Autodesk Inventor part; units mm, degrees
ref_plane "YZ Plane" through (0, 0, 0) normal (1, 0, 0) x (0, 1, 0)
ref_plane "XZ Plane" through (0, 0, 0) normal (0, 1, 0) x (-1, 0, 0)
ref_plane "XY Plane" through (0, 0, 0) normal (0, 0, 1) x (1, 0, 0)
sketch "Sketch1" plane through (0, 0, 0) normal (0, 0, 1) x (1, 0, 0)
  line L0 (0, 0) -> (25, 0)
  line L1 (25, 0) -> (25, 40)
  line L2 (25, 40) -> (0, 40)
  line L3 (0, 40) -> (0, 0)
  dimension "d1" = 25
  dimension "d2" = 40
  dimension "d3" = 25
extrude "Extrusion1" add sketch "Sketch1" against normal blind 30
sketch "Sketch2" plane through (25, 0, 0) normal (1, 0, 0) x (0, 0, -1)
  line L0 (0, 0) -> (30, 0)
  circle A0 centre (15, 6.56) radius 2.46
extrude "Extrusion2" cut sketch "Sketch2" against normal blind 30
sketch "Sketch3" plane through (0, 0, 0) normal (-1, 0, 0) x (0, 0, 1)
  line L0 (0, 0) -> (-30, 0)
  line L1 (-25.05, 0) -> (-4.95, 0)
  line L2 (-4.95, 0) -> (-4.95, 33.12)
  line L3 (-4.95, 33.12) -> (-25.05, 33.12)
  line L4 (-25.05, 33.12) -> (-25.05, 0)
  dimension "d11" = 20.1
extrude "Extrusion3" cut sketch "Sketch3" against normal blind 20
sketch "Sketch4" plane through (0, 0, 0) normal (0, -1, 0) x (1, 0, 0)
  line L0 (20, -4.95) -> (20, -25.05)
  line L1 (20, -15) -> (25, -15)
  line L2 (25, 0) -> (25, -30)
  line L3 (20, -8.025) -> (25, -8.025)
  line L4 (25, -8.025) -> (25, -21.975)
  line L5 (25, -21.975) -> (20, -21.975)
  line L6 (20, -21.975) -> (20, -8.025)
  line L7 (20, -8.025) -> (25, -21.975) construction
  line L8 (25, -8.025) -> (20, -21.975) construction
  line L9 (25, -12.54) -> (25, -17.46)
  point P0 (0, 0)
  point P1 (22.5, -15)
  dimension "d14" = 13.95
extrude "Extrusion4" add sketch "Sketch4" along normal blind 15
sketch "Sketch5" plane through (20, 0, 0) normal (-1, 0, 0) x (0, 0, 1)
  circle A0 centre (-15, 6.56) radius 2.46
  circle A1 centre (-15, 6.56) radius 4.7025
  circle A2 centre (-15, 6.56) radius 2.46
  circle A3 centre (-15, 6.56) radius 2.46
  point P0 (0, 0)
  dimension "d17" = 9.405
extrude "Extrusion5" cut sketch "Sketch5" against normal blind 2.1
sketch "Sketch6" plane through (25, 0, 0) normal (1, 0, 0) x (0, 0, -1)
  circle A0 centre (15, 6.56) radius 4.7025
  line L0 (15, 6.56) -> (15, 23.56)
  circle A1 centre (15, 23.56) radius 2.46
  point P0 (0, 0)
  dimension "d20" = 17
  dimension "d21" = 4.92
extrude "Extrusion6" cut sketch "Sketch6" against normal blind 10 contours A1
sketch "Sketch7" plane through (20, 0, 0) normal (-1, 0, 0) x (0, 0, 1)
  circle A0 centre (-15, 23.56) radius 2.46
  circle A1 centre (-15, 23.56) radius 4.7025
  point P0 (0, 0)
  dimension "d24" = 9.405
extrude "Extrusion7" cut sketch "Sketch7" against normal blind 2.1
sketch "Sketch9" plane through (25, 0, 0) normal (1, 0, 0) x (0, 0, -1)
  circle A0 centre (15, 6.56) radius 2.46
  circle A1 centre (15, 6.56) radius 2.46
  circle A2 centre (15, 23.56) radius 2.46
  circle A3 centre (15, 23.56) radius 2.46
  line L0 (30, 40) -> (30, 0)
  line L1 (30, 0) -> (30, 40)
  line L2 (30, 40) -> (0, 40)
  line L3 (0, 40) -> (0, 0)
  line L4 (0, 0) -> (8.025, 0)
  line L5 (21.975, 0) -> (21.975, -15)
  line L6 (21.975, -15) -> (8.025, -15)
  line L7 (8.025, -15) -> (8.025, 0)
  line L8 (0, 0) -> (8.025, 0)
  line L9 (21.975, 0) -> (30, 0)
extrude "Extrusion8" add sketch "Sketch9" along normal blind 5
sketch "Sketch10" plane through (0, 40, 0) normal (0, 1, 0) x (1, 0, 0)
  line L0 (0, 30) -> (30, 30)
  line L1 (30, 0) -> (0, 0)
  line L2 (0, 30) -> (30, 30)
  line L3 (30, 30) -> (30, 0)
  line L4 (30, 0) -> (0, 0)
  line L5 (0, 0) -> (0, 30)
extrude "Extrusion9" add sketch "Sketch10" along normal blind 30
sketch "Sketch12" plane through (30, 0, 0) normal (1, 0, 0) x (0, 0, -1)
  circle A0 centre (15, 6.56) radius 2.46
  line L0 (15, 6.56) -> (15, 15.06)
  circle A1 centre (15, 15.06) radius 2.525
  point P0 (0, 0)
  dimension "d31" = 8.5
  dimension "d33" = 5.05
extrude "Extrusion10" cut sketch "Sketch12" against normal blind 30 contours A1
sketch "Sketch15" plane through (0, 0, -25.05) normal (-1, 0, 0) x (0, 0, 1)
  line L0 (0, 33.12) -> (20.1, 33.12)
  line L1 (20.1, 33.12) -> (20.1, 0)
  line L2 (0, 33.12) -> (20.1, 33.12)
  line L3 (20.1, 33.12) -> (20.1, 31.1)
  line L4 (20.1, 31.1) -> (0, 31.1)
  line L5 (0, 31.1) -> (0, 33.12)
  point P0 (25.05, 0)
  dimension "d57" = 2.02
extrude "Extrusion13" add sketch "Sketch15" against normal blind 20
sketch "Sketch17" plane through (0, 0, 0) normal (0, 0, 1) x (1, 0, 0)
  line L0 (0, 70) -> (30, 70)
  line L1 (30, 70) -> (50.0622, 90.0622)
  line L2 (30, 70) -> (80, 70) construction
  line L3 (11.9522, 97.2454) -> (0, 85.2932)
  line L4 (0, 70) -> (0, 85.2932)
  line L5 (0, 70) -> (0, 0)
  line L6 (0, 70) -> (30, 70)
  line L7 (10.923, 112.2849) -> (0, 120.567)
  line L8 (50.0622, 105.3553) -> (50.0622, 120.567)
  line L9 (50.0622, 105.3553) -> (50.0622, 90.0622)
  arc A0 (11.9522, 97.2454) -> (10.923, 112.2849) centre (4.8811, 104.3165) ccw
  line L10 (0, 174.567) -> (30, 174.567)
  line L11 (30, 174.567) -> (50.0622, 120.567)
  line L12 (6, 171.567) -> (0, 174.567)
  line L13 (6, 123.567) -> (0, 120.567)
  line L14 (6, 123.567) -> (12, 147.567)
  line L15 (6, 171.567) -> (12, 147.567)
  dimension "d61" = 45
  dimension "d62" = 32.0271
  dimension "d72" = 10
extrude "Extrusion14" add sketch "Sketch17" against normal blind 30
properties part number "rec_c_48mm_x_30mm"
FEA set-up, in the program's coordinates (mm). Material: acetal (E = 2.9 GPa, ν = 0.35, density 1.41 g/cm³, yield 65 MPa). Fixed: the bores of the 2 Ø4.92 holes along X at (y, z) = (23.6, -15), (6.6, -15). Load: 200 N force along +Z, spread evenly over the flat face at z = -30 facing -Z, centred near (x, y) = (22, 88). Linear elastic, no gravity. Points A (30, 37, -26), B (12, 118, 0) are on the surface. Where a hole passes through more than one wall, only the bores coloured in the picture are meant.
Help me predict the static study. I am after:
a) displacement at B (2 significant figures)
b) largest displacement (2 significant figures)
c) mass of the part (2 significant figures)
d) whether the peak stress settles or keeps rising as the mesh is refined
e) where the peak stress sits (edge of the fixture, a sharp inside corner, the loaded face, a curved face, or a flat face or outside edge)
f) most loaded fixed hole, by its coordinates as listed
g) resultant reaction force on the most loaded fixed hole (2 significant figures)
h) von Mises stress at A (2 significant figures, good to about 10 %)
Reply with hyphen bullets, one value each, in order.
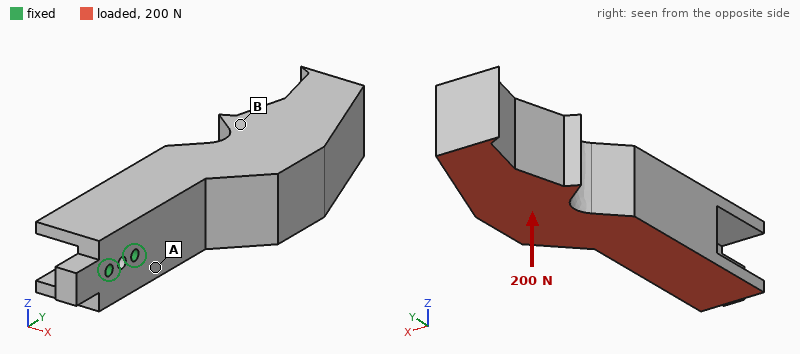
- 0.63 mm
- 1.1 mm
- 230 g
- keeps rising
- edge of the fixture
- (23.6, -15)
- 750 N
- 3.3 MPa
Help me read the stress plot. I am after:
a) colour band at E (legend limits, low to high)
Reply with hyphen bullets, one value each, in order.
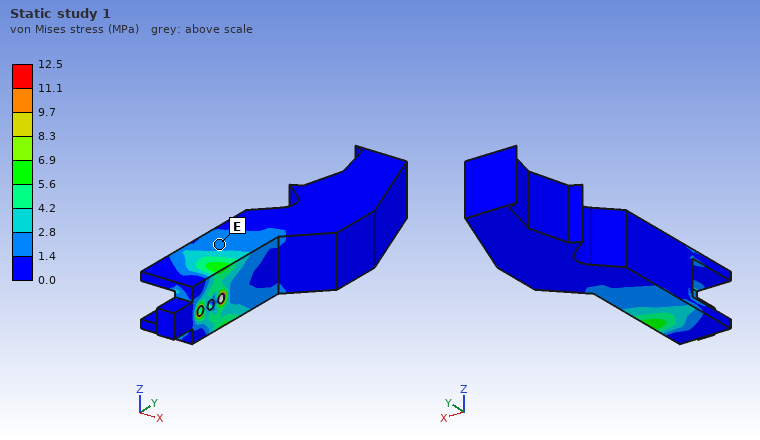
- 1.4 to 2.8 MPa
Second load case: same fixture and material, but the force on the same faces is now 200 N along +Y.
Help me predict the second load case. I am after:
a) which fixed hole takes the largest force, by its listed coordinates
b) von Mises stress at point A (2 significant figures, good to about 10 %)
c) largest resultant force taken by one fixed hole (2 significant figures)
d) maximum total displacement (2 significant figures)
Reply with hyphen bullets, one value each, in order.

- (23.6, -15)
- 1.2 MPa
- 190 N
- 0.26 mm
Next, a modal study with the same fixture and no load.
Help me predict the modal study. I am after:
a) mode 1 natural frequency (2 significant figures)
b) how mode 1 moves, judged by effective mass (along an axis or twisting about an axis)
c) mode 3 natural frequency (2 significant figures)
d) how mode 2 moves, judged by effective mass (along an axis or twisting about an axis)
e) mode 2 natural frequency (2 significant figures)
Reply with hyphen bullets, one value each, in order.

- 150 Hz
- along X
- 610 Hz
- along Z
- 170 Hz
